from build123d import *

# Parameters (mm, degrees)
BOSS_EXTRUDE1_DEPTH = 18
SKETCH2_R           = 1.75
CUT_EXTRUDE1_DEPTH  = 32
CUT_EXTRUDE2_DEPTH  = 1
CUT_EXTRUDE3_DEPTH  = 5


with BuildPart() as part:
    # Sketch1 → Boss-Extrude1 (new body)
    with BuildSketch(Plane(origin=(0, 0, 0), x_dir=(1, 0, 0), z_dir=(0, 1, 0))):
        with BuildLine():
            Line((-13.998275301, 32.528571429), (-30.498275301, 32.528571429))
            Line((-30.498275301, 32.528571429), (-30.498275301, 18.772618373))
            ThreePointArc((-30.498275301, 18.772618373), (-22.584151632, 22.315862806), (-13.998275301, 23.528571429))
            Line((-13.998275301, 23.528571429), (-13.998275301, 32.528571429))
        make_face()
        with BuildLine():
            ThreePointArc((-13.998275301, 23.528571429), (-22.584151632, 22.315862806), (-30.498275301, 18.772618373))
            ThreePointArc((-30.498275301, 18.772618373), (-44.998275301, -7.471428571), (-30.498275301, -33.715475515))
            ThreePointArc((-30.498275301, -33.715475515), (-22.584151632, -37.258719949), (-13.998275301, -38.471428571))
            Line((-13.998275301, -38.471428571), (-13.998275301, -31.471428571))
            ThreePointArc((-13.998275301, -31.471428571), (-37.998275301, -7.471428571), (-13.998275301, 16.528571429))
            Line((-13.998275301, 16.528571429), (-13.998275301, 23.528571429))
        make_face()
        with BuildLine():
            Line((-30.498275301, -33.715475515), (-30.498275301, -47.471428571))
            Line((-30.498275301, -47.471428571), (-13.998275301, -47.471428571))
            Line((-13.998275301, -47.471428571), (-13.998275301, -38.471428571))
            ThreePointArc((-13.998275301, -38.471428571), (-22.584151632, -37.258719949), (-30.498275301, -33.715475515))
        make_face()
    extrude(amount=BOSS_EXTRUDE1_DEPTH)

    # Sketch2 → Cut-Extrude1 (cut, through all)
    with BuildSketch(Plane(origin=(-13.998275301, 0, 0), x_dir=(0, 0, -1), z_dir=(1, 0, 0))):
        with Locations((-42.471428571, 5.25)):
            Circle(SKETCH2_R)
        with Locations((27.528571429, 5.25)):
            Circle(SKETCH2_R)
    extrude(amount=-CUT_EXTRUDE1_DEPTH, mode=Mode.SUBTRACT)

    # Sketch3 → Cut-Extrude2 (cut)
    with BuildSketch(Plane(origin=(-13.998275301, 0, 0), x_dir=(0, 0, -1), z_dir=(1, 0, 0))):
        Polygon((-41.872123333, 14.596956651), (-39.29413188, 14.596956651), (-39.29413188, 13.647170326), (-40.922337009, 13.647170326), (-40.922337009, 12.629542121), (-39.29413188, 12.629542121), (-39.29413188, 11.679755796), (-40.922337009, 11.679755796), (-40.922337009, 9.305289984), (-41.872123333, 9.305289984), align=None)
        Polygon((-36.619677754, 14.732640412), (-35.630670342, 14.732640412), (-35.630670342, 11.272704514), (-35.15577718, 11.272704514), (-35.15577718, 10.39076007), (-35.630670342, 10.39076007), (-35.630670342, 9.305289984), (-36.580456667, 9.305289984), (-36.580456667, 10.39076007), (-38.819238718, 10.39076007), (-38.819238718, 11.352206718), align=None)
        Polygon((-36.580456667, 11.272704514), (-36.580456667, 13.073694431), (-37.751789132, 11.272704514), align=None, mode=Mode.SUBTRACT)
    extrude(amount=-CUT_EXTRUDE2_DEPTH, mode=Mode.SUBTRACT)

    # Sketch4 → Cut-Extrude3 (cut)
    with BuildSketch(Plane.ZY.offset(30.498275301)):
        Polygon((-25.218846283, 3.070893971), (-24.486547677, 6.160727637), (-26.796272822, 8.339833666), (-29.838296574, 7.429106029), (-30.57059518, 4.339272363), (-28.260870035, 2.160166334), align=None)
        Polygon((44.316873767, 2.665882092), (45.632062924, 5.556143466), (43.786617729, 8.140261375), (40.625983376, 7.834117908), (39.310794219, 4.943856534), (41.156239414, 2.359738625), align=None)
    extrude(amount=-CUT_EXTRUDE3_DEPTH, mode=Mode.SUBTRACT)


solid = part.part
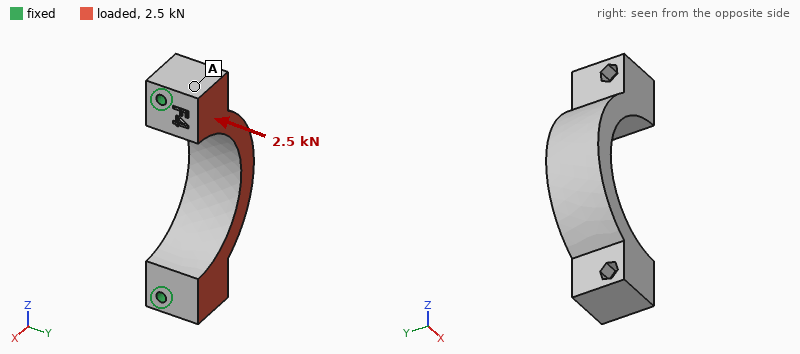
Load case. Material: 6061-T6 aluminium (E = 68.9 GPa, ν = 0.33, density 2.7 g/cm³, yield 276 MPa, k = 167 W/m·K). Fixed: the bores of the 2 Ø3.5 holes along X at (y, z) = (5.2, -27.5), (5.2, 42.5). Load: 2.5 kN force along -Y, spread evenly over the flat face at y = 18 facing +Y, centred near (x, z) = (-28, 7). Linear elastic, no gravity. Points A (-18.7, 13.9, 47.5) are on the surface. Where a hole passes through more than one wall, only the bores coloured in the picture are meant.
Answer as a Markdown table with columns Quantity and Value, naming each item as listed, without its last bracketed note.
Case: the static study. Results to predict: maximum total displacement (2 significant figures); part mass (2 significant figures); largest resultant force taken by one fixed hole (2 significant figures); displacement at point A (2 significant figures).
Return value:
| Quantity | Value |
|---|---|
| maximum total displacement | 51 µm |
| part mass | 45 g |
| largest resultant force taken by one fixed hole | 1.3 kN |
| displacement at point A | 8.3 µm |
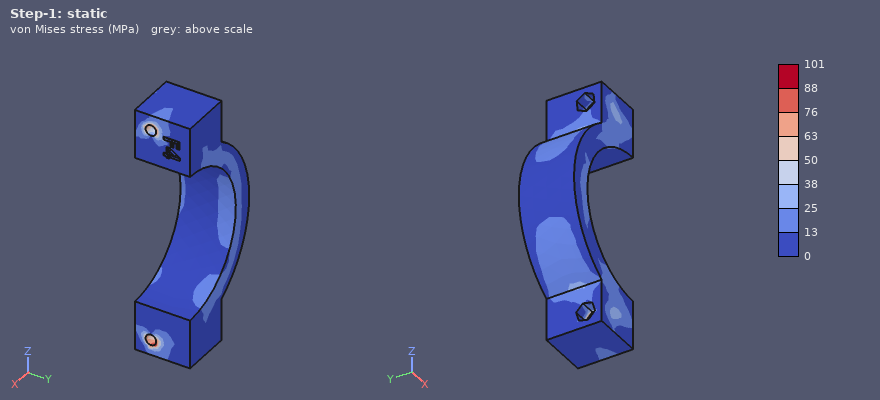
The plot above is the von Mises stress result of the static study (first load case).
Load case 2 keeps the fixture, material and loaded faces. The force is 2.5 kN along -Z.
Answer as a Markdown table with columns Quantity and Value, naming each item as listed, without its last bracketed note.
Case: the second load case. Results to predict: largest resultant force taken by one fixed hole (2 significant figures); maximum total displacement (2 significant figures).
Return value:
| Quantity | Value |
|---|---|
| largest resultant force taken by one fixed hole | 1.3 kN |
| maximum total displacement | 14 µm |
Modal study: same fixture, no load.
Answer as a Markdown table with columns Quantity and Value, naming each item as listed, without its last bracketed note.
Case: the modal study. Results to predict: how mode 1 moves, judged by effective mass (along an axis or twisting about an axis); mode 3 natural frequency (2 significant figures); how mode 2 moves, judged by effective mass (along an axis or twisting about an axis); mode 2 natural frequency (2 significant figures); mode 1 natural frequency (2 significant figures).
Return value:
| Quantity | Value |
|---|---|
| how mode 1 moves, judged by effective mass | along Y |
| mode 3 natural frequency | 17 kHz |
| how mode 2 moves, judged by effective mass | along Z |
| mode 2 natural frequency | 13 kHz |
| mode 1 natural frequency | 6400 Hz |
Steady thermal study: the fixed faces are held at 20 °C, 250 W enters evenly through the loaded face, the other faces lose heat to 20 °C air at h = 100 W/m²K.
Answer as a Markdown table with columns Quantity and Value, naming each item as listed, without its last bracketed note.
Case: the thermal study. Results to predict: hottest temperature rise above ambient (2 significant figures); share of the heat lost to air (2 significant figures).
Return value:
| Quantity | Value |
|---|---|
| hottest temperature rise above ambient | 76 K |
| share of the heat lost to air | 7.5 % |
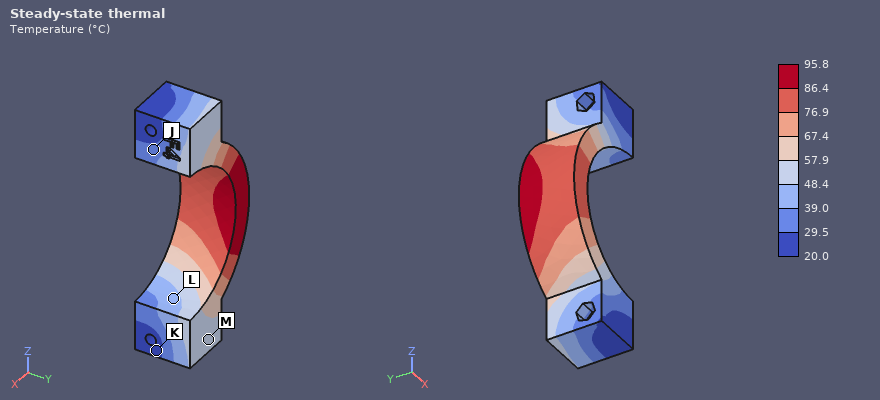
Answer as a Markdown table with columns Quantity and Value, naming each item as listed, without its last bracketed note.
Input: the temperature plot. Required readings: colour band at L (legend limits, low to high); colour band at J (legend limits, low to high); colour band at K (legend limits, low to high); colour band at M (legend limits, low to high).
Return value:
| Quantity | Value |
|---|---|
| colour band at L | 39.0 to 48.4 °C |
| colour band at J | 29.5 to 39.0 °C |
| colour band at K | 20.0 to 29.5 °C |
| colour band at M | 48.4 to 57.9 °C |
